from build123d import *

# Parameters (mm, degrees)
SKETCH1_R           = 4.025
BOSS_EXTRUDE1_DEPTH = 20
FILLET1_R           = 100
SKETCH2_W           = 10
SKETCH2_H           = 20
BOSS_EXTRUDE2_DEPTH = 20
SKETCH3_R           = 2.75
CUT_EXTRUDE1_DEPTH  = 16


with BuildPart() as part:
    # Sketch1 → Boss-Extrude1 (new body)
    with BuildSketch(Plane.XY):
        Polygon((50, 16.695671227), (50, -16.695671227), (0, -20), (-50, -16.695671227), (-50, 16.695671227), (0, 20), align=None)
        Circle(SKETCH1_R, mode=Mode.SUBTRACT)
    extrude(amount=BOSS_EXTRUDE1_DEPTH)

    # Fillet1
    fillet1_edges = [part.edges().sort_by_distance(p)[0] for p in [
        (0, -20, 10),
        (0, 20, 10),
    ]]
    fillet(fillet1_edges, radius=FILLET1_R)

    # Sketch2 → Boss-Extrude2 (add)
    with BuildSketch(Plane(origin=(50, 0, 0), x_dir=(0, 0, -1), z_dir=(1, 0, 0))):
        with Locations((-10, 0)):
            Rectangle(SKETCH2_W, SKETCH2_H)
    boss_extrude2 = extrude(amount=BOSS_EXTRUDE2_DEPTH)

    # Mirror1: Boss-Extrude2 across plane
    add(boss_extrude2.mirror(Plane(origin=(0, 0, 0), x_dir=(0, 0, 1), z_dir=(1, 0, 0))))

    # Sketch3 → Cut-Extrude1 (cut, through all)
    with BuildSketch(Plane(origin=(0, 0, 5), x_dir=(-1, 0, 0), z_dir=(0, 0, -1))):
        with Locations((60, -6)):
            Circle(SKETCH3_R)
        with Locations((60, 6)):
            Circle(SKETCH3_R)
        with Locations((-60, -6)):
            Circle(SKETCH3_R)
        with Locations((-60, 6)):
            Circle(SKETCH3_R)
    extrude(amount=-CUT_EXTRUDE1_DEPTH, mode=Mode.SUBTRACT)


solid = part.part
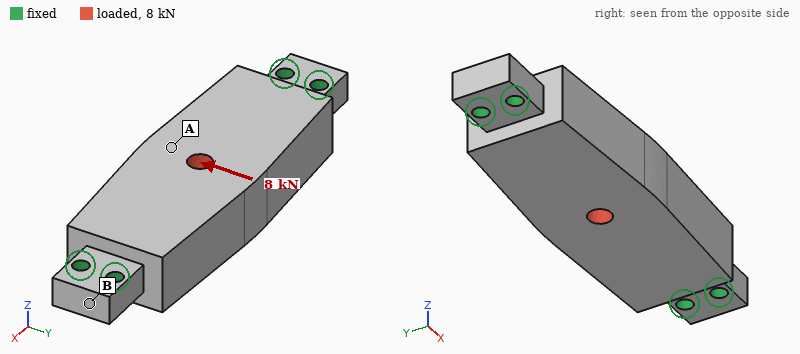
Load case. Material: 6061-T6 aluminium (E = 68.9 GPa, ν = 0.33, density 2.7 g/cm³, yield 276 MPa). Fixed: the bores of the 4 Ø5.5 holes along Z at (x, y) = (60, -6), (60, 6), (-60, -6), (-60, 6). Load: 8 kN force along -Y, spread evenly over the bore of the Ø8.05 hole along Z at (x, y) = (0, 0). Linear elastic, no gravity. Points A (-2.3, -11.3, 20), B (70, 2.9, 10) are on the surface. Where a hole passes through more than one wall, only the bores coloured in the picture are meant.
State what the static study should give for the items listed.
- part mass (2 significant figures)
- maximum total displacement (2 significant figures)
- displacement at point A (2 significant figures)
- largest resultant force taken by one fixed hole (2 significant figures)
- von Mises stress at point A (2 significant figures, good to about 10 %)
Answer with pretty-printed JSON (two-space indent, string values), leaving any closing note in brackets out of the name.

{
  "part mass": "210 g",
  "maximum total displacement": "47 µm",
  "displacement at point A": "45 µm",
  "largest resultant force taken by one fixed hole": "3.8 kN",
  "von Mises stress at point A": "22 MPa"
}
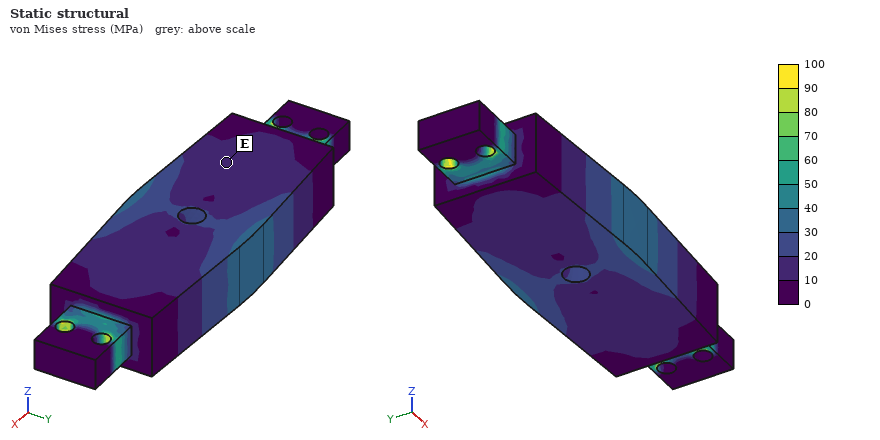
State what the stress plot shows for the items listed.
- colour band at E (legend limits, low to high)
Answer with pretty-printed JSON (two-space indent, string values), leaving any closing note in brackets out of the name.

{
  "colour band at E": "10 to 20 MPa"
}
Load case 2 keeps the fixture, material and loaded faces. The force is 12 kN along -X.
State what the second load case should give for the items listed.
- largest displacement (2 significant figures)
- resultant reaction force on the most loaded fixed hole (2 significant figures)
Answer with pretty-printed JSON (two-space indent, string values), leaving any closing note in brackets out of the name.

{
  "largest displacement": "13 µm",
  "resultant reaction force on the most loaded fixed hole": "3.0 kN"
}
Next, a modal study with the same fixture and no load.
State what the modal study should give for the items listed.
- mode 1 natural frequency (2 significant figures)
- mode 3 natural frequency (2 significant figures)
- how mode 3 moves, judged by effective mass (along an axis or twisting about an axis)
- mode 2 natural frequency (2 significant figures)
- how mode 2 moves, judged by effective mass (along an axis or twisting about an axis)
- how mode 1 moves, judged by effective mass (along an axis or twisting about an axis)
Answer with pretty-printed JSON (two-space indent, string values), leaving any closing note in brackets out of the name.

{
  "mode 1 natural frequency": "3900 Hz",
  "mode 3 natural frequency": "6200 Hz",
  "how mode 3 moves, judged by effective mass": "along Y",
  "mode 2 natural frequency": "5000 Hz",
  "how mode 2 moves, judged by effective mass": "twisting about X",
  "how mode 1 moves, judged by effective mass": "along Z"
}
